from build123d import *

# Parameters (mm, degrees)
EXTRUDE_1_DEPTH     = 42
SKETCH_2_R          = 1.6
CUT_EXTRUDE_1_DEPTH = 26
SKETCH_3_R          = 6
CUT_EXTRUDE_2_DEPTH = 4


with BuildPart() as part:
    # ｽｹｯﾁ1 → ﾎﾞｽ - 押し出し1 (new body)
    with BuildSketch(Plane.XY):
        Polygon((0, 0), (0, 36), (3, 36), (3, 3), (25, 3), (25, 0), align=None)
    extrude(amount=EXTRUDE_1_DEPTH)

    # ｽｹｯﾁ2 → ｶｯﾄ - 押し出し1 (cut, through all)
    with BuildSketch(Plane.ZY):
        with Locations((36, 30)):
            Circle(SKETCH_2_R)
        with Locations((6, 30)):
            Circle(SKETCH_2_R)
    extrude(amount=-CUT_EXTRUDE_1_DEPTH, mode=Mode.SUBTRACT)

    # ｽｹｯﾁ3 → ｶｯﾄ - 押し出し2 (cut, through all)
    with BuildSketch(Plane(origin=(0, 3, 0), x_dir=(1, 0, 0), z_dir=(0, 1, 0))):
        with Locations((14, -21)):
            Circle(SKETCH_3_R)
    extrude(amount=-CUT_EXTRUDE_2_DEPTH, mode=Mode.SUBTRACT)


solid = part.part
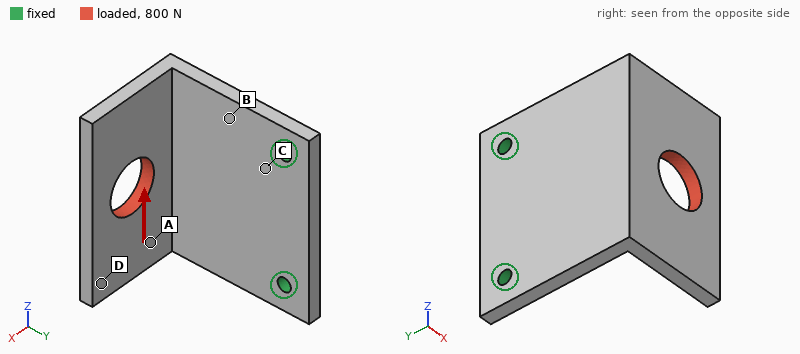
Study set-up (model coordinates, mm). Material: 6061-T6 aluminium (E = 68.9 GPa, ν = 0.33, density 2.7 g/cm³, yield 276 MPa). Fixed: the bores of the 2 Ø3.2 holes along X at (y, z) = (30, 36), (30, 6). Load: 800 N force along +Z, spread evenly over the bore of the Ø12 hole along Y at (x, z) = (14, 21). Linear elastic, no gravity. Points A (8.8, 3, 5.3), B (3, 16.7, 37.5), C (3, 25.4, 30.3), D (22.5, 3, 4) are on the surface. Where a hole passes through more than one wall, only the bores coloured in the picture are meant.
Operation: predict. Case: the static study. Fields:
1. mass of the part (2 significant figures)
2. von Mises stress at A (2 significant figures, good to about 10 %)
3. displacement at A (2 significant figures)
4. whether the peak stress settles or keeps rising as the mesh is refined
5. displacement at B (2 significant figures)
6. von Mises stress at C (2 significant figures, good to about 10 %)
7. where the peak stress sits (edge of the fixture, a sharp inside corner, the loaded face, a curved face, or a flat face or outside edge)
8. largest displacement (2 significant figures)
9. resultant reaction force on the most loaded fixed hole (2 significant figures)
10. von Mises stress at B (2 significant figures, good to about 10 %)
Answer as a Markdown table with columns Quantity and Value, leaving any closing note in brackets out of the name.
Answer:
| Quantity | Value |
|---|---|
| mass of the part | 19 g |
| von Mises stress at A | 55 MPa |
| displacement at A | 0.27 mm |
| whether the peak stress settles or keeps rising as the mesh is refined | keeps rising |
| displacement at B | 0.094 mm |
| von Mises stress at C | 78 MPa |
| where the peak stress sits | edge of the fixture |
| largest displacement | 0.51 mm |
| resultant reaction force on the most loaded fixed hole | 880 N |
| von Mises stress at B | 93 MPa |
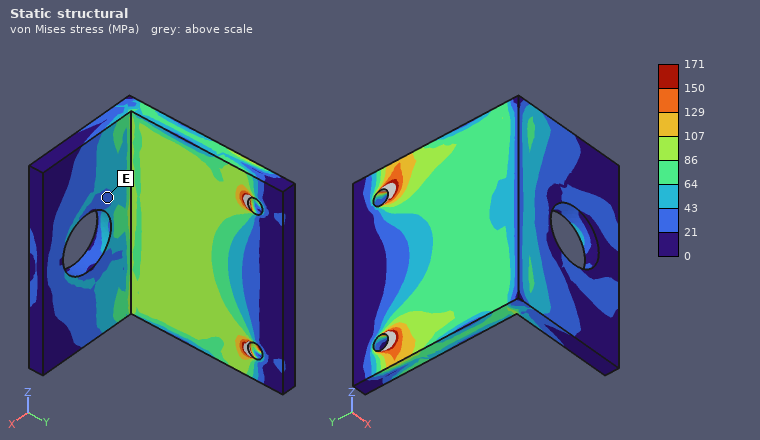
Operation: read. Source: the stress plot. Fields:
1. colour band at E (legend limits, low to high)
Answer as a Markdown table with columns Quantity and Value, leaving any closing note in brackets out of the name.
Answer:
| Quantity | Value |
|---|---|
| colour band at E | 21 to 43 MPa |
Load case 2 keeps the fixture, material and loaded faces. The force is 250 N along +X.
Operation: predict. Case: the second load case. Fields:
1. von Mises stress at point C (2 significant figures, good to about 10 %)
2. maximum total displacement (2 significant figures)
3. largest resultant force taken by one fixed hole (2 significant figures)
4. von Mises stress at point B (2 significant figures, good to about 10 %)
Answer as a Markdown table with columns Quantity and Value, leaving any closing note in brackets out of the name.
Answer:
| Quantity | Value |
|---|---|
| von Mises stress at point C | 80 MPa |
| maximum total displacement | 0.53 mm |
| largest resultant force taken by one fixed hole | 130 N |
| von Mises stress at point B | 61 MPa |
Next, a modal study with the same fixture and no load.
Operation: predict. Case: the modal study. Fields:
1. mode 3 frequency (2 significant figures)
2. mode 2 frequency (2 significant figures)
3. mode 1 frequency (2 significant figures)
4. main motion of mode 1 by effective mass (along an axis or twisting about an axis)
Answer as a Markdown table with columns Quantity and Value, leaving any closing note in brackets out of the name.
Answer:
| Quantity | Value |
|---|---|
| mode 3 frequency | 3600 Hz |
| mode 2 frequency | 2300 Hz |
| mode 1 frequency | 1200 Hz |
| main motion of mode 1 by effective mass | along X |
